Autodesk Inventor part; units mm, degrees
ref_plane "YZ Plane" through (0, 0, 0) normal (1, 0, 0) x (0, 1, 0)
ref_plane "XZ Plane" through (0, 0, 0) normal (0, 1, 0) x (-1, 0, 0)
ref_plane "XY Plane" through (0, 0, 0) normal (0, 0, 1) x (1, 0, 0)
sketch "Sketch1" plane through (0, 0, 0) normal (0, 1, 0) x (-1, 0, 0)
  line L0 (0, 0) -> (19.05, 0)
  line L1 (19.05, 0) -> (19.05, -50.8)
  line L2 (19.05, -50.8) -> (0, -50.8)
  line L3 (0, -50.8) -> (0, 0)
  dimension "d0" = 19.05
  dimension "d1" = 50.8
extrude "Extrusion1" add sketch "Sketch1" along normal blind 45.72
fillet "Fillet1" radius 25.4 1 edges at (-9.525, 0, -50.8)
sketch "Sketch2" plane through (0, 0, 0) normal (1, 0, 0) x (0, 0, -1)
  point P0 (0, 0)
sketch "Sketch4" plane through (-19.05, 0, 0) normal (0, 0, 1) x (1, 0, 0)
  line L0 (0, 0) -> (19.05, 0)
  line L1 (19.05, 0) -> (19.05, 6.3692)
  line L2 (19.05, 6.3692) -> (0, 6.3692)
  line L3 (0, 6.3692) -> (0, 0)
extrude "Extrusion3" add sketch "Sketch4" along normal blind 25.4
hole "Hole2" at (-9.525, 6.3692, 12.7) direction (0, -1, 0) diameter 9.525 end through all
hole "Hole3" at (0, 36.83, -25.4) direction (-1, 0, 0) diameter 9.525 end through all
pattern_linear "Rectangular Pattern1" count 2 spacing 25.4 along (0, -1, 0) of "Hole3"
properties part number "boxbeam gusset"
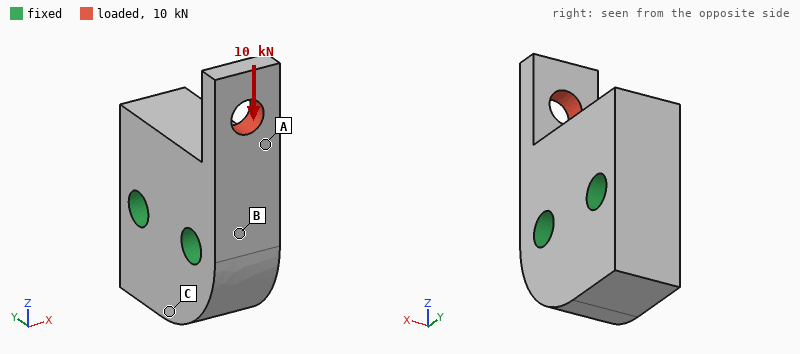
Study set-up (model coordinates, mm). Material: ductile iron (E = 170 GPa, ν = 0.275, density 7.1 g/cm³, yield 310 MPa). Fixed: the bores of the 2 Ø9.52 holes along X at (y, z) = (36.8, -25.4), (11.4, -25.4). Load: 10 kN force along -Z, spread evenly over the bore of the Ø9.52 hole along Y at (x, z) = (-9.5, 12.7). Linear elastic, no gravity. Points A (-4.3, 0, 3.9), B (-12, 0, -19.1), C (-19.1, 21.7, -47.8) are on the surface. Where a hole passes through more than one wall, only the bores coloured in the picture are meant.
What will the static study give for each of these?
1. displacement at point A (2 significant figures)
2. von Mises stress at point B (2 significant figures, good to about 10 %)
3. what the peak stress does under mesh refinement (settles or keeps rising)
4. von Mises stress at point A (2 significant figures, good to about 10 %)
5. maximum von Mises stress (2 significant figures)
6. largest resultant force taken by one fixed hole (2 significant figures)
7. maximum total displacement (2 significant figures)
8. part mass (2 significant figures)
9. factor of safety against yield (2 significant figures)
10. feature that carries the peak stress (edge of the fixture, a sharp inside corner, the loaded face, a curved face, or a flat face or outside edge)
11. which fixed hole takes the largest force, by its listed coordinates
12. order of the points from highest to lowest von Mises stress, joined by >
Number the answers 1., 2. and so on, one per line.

1. 16 µm
2. 37 MPa
3. settles
4. 93 MPa
5. 210 MPa
6. 12 kN
7. 34 µm
8. 290 g
9. 1.5
10. the loaded face
11. (11.4, -25.4)
12. A > B > C
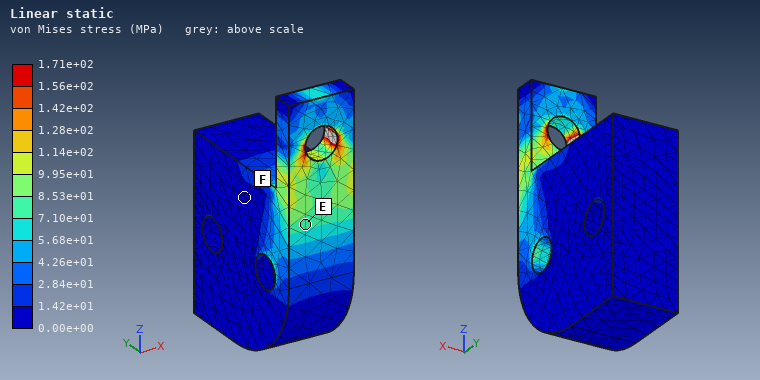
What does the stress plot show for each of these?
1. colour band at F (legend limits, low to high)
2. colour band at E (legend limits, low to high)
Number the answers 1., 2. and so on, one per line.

1. 0.00e+00 to 1.42e+01 MPa
2. 7.10e+01 to 8.53e+01 MPa
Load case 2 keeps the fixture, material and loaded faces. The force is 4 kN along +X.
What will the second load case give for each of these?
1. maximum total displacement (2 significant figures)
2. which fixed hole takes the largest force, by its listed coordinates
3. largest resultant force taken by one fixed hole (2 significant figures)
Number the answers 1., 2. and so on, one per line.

1. 91 µm
2. (11.4, -25.4)
3. 3.9 kN
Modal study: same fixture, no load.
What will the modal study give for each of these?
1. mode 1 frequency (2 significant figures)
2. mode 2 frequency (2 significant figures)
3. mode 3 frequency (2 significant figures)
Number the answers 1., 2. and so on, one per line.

1. 5600 Hz
2. 8600 Hz
3. 14 kHz
